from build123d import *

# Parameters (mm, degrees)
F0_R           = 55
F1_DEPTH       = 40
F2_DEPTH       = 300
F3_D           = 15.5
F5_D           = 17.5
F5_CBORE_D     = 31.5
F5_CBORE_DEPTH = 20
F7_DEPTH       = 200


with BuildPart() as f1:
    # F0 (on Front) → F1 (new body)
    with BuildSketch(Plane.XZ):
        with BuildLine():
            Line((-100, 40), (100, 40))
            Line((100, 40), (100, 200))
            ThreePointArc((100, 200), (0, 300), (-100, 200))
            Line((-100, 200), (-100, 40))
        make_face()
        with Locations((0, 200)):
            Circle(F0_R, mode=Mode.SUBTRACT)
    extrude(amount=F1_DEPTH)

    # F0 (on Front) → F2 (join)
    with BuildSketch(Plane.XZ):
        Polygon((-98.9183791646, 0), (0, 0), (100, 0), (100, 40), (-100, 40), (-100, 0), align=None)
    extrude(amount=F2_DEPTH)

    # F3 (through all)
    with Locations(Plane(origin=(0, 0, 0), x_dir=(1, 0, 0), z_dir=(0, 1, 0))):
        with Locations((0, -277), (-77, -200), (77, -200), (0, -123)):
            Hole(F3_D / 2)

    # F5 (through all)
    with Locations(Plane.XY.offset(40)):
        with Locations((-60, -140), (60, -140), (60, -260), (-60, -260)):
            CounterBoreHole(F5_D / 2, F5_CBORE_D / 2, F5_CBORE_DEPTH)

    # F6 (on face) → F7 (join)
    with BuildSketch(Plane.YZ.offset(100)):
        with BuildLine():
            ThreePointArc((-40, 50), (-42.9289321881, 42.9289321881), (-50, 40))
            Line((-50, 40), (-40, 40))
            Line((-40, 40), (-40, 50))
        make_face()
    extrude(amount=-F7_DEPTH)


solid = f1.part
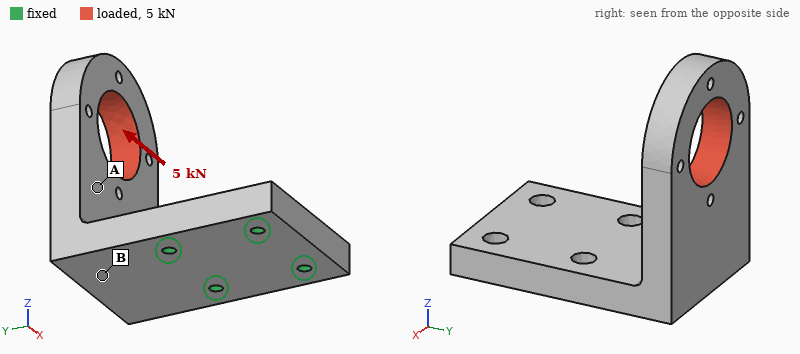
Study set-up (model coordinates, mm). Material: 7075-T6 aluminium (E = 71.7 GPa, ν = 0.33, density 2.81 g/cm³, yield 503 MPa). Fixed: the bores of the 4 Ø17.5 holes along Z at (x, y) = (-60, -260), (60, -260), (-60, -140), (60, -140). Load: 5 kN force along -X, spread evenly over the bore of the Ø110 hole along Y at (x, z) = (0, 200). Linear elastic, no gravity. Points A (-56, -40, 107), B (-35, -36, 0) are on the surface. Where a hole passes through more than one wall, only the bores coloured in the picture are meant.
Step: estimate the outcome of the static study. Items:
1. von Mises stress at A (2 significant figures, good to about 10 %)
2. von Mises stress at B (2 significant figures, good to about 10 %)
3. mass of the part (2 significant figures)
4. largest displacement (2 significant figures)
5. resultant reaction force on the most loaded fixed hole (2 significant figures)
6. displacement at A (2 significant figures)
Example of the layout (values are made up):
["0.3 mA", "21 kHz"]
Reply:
["2.6 MPa", "7.4 MPa", "11 kg", "0.20 mm", "9.8 kN", "0.072 mm"]
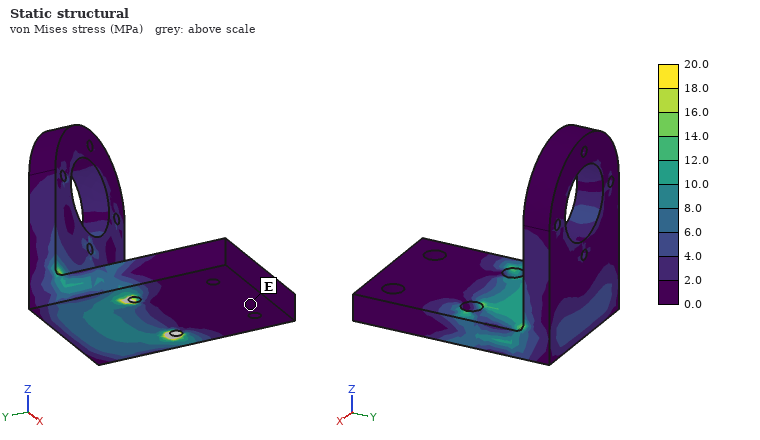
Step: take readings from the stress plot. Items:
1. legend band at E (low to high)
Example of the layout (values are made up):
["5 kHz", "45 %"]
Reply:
["0.0 to 2.0 MPa"]
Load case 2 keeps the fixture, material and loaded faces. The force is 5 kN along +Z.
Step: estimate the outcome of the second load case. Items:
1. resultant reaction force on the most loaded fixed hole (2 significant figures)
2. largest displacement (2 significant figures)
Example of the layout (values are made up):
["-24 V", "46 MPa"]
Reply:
["5.2 kN", "0.21 mm"]
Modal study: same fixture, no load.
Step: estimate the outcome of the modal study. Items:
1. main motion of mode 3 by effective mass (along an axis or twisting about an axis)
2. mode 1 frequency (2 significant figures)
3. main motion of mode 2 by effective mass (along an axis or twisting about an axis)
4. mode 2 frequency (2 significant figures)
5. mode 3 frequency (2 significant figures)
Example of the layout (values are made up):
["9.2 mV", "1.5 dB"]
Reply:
["along Z", "300 Hz", "along X", "540 Hz", "900 Hz"]
